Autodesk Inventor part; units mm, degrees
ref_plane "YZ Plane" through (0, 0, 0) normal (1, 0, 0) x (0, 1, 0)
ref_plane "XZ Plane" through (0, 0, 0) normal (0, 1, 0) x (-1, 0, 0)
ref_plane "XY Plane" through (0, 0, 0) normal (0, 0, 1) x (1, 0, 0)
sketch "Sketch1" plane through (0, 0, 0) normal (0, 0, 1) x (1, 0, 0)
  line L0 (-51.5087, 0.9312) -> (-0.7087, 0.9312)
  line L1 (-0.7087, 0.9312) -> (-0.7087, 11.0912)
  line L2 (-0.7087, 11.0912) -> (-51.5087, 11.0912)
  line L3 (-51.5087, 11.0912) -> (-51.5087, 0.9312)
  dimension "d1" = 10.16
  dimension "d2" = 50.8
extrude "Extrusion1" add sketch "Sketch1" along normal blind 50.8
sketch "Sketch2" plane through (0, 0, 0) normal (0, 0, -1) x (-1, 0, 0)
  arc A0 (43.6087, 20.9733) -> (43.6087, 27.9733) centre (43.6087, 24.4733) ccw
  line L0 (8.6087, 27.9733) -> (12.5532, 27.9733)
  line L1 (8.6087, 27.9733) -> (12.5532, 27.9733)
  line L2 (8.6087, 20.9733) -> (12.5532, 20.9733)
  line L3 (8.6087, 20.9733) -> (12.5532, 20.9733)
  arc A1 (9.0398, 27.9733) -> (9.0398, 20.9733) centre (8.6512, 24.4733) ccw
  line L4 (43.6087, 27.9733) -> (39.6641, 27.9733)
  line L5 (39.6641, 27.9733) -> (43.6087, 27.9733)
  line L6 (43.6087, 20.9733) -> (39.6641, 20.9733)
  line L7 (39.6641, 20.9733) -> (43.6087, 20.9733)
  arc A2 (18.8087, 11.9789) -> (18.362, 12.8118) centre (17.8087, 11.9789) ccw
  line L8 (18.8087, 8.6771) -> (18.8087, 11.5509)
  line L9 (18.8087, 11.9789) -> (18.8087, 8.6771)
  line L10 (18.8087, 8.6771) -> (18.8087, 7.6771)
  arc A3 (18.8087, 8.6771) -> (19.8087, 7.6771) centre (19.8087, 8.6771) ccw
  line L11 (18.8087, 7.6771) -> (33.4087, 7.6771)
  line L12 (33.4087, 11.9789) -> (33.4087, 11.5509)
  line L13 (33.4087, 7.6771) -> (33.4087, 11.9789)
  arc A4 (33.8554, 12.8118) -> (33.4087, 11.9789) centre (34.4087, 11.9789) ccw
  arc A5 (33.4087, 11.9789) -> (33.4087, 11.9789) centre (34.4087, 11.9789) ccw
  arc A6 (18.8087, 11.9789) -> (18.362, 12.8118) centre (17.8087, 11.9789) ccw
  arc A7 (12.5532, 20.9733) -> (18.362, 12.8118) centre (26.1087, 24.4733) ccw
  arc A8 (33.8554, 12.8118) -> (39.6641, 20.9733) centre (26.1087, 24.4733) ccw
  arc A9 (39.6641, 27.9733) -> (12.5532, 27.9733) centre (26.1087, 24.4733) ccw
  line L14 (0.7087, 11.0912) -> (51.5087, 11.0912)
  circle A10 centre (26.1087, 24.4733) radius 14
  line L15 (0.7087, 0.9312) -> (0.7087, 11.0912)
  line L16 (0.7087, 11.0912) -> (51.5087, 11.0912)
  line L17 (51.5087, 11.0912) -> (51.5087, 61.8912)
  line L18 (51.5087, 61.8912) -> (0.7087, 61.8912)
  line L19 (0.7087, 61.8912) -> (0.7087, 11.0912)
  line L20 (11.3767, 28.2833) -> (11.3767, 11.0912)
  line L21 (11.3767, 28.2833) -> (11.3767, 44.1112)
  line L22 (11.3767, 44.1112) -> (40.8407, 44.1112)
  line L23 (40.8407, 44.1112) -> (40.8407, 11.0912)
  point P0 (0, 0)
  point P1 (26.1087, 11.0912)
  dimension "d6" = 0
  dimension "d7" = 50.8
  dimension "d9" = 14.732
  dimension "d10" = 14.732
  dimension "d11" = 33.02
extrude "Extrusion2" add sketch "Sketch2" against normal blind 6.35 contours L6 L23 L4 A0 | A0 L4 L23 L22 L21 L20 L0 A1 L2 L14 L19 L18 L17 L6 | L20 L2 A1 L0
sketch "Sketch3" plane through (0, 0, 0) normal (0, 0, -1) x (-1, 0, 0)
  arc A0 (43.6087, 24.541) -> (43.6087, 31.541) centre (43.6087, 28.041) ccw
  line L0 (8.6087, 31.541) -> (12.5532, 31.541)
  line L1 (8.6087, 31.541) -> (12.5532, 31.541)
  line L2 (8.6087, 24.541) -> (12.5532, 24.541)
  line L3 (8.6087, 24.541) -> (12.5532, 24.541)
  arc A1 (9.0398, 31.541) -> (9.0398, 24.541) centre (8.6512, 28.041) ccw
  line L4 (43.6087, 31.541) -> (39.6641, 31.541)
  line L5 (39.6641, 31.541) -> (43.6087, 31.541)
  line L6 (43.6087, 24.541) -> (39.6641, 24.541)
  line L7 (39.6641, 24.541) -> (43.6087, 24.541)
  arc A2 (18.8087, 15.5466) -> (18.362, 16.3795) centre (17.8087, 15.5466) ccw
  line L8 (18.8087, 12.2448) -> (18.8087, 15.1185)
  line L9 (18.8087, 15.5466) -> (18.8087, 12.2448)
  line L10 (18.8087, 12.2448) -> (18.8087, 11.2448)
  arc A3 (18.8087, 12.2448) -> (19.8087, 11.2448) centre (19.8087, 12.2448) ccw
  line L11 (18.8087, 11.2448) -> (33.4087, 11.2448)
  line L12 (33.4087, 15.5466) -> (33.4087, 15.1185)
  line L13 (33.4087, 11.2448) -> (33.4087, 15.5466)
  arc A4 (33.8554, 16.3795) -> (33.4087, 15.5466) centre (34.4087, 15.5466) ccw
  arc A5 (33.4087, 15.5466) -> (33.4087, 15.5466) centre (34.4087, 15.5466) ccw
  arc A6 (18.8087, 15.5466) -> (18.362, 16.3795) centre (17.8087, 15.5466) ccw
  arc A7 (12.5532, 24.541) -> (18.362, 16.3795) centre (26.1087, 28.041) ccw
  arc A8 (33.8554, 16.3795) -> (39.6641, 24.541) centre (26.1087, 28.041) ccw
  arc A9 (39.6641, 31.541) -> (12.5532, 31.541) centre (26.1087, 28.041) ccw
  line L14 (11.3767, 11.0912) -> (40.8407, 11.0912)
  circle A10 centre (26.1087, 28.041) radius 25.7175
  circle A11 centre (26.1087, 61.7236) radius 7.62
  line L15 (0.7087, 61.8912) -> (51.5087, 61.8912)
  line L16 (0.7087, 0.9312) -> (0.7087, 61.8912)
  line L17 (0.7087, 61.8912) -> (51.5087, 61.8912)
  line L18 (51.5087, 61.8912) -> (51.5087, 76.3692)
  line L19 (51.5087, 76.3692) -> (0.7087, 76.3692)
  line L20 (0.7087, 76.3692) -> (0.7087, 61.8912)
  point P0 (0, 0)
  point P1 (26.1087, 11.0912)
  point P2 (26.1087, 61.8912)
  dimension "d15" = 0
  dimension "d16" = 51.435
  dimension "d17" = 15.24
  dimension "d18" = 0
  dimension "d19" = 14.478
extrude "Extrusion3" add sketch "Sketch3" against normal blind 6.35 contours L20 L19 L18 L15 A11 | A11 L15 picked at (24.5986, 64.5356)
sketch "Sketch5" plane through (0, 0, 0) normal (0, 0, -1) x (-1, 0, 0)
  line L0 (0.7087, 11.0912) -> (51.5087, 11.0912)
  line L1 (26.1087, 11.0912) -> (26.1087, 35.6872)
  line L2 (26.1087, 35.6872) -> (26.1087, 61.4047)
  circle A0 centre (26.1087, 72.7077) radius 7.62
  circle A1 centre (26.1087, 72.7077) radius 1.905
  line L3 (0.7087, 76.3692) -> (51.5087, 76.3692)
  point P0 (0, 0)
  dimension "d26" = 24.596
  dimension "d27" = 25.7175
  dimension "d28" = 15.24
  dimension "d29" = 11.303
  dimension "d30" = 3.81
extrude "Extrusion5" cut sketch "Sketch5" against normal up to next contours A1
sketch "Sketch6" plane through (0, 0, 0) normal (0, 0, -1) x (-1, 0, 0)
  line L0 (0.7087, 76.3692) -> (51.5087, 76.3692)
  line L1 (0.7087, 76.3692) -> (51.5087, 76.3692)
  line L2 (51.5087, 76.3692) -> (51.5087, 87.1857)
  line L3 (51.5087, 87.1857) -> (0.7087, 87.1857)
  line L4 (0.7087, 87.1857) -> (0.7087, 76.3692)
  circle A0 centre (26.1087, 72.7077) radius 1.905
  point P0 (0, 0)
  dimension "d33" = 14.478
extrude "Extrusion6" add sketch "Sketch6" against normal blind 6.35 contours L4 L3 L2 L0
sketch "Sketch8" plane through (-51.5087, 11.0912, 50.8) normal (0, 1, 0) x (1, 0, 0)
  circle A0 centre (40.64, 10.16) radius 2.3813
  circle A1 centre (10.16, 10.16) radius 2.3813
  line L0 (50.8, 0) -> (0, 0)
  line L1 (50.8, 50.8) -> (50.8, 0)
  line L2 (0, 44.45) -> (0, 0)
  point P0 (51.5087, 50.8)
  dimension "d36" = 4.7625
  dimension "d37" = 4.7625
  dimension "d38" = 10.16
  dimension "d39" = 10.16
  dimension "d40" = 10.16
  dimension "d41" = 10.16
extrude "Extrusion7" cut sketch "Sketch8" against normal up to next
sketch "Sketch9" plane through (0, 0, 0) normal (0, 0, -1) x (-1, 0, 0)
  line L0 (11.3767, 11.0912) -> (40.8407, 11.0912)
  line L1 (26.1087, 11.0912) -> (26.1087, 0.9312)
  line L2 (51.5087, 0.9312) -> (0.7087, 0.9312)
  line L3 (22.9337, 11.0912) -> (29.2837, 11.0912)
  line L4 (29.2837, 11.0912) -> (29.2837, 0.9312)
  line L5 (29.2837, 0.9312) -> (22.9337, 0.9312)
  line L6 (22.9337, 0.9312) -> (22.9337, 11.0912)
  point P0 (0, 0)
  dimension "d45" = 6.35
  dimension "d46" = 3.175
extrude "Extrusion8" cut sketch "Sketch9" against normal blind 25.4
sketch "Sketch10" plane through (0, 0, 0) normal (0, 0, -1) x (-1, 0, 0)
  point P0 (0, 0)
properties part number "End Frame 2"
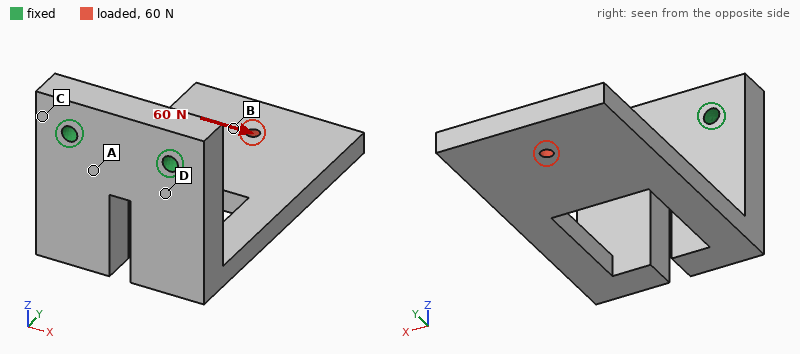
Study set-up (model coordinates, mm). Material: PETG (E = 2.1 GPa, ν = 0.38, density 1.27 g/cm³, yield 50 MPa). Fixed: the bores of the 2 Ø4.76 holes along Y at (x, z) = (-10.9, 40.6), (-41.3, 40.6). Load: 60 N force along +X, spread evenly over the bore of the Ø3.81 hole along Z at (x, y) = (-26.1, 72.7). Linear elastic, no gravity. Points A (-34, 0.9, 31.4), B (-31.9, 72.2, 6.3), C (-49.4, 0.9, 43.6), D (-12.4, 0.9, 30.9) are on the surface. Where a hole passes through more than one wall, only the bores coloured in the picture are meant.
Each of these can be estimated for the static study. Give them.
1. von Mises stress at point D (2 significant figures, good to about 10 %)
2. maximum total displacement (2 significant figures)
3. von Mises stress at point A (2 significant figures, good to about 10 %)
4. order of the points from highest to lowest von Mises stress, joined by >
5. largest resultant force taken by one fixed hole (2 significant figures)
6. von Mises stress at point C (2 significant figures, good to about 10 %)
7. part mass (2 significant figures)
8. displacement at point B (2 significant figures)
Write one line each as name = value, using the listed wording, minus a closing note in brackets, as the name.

von Mises stress at point D = 4.2 MPa
maximum total displacement = 1.3 mm
von Mises stress at point A = 3.3 MPa
order of the points from highest to lowest von Mises stress, joined by > = D > A > C > B
largest resultant force taken by one fixed hole = 130 N
von Mises stress at point C = 1.8 MPa
part mass = 54 g
displacement at point B = 1.0 mm
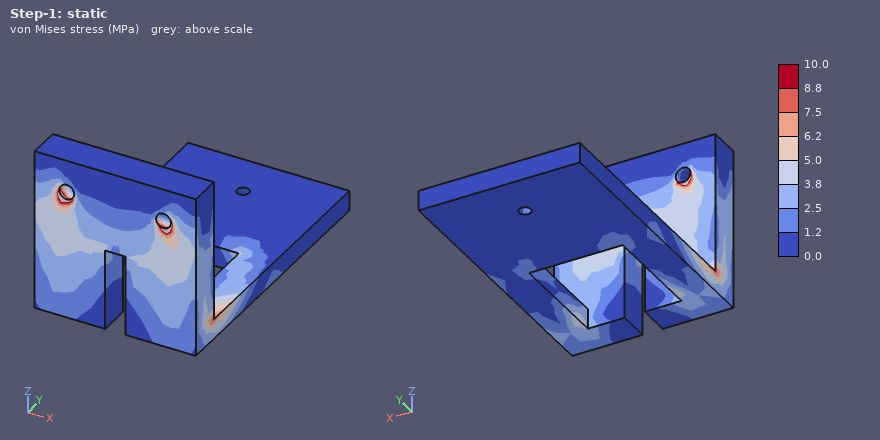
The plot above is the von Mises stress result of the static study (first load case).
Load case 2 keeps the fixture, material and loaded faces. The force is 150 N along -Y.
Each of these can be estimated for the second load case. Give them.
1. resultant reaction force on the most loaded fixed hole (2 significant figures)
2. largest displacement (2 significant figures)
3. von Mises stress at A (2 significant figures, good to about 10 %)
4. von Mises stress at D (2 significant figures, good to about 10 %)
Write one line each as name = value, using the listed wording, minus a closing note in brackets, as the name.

resultant reaction force on the most loaded fixed hole = 75 N
largest displacement = 1.2 mm
von Mises stress at A = 4.0 MPa
von Mises stress at D = 5.2 MPa
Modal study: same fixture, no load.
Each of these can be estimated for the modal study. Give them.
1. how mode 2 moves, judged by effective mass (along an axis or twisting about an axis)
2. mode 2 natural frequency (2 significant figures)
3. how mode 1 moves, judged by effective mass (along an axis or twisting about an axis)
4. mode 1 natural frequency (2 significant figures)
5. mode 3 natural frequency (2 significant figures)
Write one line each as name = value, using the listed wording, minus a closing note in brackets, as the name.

how mode 2 moves, judged by effective mass = along X
mode 2 natural frequency = 300 Hz
how mode 1 moves, judged by effective mass = along Z
mode 1 natural frequency = 130 Hz
mode 3 natural frequency = 520 Hz
